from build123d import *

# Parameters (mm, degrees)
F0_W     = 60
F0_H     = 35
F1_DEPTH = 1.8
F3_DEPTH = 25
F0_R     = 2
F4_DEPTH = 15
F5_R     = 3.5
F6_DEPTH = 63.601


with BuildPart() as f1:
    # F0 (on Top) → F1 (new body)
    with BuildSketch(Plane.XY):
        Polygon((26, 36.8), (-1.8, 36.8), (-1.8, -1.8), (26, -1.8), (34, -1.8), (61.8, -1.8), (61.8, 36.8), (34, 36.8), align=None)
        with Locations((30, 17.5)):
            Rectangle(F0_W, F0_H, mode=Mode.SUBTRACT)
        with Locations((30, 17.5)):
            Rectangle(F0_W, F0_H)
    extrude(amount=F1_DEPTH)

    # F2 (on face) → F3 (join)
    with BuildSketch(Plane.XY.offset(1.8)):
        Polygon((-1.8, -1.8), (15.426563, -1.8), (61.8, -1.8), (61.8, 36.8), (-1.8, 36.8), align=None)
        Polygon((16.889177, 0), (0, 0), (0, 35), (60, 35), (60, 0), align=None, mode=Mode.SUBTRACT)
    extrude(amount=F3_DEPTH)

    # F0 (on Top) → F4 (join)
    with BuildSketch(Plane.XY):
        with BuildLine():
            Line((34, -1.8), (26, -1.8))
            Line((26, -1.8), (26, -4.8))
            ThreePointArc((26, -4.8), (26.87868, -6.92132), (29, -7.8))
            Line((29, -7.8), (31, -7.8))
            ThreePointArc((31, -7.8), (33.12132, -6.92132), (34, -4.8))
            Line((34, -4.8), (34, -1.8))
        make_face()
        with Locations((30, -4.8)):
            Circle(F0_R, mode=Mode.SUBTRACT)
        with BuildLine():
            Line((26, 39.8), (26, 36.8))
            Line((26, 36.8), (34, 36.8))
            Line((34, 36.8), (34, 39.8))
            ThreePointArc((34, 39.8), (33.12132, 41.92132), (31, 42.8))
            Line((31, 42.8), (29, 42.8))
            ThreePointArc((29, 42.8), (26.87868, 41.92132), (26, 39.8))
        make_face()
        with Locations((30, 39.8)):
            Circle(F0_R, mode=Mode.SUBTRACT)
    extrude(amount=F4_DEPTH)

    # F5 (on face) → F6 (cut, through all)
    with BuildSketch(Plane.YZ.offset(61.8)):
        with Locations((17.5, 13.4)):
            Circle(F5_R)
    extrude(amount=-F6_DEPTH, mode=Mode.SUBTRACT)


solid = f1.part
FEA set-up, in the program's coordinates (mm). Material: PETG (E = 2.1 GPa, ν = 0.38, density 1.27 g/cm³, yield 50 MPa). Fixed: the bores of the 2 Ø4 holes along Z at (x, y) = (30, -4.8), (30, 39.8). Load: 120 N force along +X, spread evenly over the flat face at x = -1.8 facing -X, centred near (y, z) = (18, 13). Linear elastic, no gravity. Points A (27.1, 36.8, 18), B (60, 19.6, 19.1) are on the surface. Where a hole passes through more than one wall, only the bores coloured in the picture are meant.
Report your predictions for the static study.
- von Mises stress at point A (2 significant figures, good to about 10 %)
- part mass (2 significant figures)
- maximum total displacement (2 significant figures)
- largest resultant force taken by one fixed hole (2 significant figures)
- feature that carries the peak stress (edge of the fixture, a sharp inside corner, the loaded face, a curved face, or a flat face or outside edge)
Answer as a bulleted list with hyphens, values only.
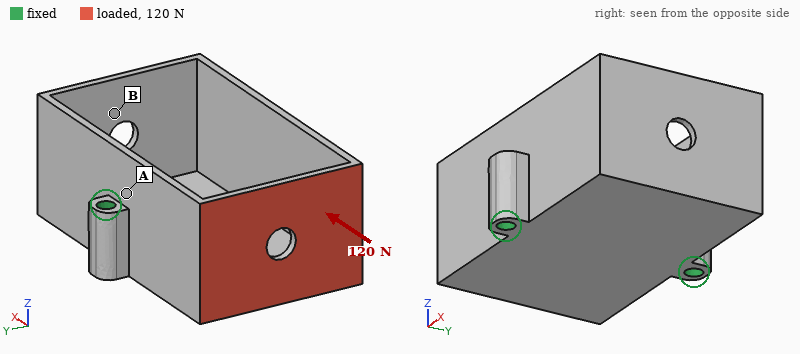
- 4.2 MPa
- 18 g
- 0.95 mm
- 61 N
- the loaded face
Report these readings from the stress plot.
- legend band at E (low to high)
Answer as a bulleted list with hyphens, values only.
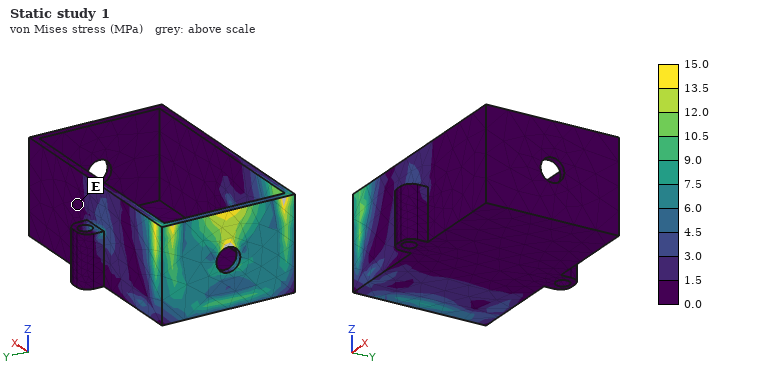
- 0.0 to 1.5 MPa
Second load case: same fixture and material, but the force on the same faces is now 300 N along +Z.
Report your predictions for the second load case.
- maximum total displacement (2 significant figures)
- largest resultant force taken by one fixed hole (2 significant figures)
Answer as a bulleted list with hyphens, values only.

- 0.95 mm
- 150 N
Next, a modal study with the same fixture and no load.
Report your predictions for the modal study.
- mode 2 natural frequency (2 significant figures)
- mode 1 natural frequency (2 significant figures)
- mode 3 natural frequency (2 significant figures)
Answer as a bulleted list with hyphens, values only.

- 1300 Hz
- 1100 Hz
- 1500 Hz
